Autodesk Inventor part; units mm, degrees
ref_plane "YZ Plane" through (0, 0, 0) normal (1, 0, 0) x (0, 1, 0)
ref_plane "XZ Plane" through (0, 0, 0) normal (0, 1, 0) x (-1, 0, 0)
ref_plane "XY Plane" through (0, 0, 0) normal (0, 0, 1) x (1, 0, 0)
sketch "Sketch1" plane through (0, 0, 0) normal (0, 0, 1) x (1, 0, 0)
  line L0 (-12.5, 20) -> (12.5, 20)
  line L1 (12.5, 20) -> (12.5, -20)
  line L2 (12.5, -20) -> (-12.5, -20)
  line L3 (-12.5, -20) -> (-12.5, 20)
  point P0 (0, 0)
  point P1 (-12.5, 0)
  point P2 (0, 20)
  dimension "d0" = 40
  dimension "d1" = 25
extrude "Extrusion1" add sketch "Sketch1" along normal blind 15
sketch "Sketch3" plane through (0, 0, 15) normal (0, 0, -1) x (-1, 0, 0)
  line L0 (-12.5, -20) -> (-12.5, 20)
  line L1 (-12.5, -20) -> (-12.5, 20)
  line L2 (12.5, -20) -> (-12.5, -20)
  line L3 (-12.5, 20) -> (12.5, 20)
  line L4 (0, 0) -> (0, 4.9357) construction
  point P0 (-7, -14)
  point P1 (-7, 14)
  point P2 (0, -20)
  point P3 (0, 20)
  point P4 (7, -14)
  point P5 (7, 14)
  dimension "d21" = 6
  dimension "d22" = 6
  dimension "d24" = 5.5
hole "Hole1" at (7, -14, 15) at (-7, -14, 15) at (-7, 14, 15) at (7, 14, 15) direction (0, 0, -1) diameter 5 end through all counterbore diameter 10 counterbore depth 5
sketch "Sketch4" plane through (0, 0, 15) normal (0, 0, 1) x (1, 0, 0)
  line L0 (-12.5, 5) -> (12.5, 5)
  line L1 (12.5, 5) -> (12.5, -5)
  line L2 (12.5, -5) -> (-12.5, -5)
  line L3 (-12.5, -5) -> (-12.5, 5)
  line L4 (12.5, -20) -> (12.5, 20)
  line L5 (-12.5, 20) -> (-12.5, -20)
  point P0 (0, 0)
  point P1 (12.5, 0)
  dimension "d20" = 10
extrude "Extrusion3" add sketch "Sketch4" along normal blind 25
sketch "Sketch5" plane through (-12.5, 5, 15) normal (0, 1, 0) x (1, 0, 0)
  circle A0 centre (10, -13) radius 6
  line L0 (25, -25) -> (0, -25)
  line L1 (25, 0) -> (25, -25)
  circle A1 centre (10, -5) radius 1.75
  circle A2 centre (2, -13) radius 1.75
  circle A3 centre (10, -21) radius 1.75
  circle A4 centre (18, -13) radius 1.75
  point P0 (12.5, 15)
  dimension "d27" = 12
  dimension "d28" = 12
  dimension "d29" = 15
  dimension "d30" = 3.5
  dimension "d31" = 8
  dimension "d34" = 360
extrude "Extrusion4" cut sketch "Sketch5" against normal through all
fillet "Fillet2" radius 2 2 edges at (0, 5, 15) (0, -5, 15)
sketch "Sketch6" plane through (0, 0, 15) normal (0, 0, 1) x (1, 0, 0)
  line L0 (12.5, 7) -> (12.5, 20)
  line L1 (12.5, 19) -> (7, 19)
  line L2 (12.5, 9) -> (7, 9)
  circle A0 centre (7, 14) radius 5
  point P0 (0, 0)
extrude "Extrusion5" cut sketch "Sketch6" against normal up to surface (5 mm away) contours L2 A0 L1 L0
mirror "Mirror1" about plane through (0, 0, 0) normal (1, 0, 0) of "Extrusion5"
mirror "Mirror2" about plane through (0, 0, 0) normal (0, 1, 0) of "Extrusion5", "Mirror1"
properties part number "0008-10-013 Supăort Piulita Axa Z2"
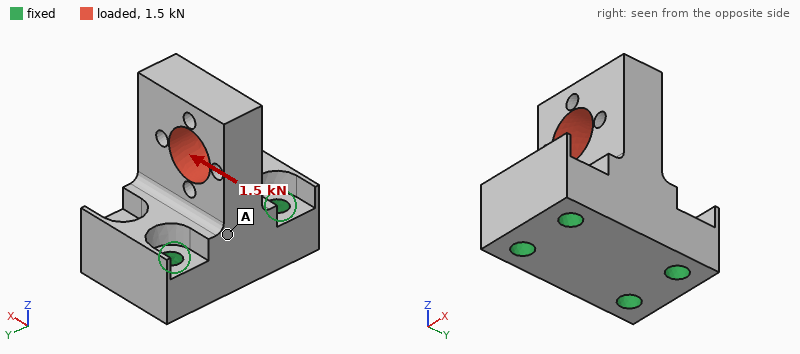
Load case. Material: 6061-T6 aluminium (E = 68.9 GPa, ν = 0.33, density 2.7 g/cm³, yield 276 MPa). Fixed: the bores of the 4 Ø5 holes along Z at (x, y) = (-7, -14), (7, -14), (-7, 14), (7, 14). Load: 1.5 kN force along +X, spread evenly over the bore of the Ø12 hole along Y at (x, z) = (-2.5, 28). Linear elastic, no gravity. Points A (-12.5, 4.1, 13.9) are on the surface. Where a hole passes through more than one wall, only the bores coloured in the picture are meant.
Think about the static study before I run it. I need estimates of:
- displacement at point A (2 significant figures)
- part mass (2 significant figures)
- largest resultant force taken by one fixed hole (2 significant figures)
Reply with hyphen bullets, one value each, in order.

- 7.3 µm
- 46 g
- 1.1 kN
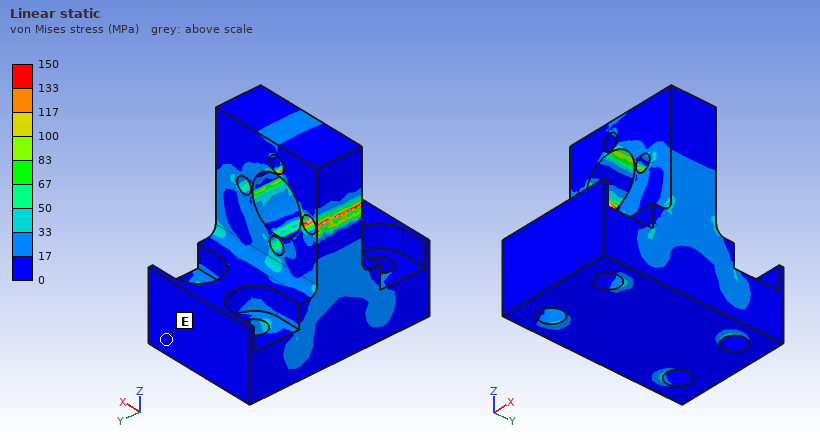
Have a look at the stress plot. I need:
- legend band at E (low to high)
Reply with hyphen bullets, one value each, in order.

- 0 to 17 MPa
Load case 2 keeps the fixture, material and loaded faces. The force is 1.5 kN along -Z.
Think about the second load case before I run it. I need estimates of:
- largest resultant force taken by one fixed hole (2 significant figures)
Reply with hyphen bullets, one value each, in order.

- 510 N
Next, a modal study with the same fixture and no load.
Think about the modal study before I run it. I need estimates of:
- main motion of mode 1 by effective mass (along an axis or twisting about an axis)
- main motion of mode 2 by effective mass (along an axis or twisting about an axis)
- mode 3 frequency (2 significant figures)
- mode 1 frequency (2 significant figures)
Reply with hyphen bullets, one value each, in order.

- along Y
- along X
- 16 kHz
- 8600 Hz
